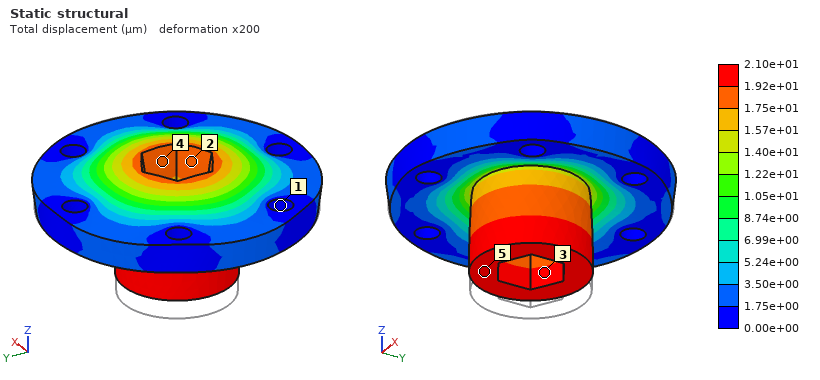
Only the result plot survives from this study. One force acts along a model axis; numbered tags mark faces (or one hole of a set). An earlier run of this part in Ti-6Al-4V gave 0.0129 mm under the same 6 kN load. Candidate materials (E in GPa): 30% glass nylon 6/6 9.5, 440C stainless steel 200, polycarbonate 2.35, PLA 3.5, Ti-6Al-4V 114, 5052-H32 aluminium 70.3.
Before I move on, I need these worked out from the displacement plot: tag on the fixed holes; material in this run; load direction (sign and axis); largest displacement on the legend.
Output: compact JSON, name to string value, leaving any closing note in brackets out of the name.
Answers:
{"tag on the fixed holes": "1", "material in this run": "5052-H32 aluminium", "load direction": "+Z", "largest displacement on the legend": "2.10e+01 µm"}
